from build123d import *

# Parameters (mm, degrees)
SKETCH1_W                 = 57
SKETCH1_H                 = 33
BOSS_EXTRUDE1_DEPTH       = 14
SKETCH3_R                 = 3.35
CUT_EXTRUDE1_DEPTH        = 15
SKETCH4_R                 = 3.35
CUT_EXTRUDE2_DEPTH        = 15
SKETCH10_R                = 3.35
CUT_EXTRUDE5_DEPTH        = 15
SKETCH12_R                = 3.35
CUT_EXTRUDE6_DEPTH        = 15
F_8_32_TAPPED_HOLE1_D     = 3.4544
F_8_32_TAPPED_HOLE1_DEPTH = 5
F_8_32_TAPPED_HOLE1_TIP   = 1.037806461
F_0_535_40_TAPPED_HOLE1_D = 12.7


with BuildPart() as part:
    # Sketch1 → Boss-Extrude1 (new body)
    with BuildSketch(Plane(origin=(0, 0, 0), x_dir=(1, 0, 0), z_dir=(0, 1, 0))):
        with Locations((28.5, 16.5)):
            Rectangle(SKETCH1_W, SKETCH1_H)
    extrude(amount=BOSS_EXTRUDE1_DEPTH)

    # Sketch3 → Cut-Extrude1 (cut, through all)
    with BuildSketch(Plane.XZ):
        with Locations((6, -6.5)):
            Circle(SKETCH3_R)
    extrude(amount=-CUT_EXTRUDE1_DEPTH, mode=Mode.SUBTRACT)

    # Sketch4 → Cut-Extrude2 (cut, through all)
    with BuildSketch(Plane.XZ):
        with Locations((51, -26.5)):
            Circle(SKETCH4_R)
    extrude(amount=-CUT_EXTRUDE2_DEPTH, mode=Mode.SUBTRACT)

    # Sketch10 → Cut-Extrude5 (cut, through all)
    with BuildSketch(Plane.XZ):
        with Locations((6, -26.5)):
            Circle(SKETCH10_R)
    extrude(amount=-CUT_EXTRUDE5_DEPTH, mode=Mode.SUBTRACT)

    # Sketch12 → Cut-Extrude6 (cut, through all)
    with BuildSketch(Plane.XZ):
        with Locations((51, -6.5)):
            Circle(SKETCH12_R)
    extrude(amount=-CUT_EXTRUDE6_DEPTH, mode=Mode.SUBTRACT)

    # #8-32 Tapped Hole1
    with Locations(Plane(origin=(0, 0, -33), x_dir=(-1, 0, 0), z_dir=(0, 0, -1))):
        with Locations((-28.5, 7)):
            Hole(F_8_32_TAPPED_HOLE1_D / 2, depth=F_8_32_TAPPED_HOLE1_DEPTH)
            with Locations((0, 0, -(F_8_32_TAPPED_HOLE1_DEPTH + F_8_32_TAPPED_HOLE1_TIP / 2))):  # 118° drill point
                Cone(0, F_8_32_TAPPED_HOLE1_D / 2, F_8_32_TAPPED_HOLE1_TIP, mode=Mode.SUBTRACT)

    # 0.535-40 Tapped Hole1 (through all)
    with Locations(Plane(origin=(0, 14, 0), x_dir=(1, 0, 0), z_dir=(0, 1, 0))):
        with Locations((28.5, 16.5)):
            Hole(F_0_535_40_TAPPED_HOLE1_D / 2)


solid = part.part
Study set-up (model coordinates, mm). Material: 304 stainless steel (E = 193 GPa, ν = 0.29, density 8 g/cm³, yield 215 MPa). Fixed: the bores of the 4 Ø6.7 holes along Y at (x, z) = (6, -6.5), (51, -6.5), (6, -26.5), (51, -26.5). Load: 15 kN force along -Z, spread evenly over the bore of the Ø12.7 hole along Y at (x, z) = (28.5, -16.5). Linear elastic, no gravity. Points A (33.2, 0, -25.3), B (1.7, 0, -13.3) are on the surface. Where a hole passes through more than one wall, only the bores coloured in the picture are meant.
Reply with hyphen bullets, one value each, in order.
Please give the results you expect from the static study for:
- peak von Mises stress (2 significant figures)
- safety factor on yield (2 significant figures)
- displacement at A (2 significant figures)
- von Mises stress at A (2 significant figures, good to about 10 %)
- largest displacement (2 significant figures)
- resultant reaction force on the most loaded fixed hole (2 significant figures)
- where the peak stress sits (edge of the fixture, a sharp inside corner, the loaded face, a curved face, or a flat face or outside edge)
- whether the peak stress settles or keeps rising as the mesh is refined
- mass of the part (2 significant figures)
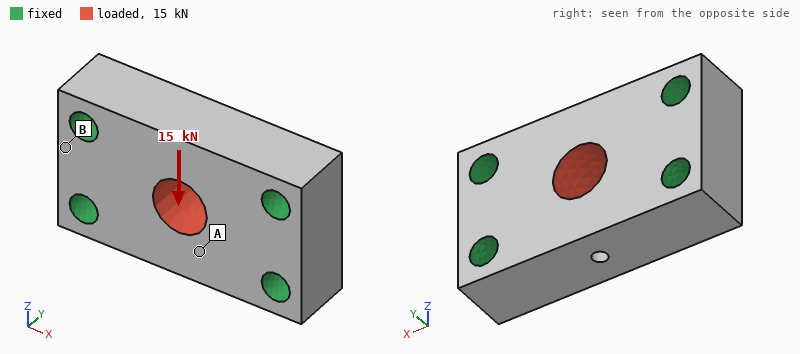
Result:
- 88 MPa
- 2.4
- 4.7 µm
- 31 MPa
- 5.8 µm
- 4.8 kN
- a curved face
- settles
- 180 g
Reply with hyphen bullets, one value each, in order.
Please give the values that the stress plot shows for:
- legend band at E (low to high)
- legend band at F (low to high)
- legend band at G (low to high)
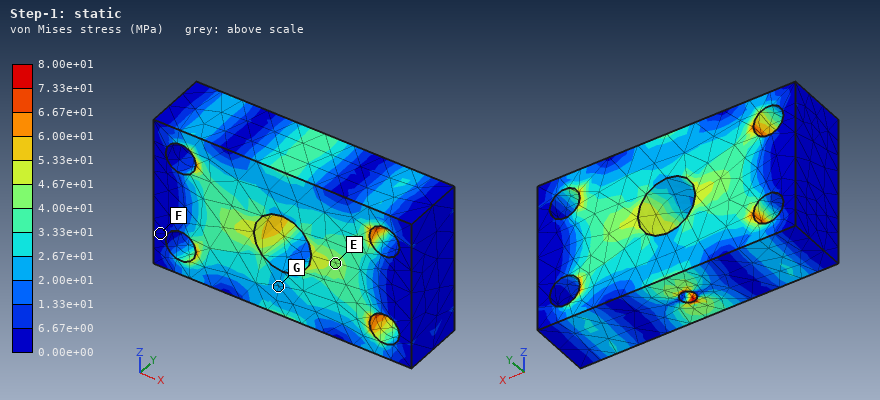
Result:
- 4.00e+01 to 4.67e+01 MPa
- 0.00e+00 to 6.67e+00 MPa
- 2.00e+01 to 2.67e+01 MPa
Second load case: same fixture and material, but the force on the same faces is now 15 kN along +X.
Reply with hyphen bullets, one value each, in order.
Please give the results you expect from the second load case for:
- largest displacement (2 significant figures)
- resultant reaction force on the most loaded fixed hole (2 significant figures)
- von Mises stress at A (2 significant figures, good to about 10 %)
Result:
- 2.2 µm
- 3.9 kN
- 17 MPa
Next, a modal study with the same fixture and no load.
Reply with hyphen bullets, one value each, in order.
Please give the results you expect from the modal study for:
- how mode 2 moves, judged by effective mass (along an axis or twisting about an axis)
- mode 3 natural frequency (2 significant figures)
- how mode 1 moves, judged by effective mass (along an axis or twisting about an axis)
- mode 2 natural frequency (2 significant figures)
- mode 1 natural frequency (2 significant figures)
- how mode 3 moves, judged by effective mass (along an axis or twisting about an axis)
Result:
- twisting about X
- 34 kHz
- along Y
- 31 kHz
- 27 kHz
- along Z
